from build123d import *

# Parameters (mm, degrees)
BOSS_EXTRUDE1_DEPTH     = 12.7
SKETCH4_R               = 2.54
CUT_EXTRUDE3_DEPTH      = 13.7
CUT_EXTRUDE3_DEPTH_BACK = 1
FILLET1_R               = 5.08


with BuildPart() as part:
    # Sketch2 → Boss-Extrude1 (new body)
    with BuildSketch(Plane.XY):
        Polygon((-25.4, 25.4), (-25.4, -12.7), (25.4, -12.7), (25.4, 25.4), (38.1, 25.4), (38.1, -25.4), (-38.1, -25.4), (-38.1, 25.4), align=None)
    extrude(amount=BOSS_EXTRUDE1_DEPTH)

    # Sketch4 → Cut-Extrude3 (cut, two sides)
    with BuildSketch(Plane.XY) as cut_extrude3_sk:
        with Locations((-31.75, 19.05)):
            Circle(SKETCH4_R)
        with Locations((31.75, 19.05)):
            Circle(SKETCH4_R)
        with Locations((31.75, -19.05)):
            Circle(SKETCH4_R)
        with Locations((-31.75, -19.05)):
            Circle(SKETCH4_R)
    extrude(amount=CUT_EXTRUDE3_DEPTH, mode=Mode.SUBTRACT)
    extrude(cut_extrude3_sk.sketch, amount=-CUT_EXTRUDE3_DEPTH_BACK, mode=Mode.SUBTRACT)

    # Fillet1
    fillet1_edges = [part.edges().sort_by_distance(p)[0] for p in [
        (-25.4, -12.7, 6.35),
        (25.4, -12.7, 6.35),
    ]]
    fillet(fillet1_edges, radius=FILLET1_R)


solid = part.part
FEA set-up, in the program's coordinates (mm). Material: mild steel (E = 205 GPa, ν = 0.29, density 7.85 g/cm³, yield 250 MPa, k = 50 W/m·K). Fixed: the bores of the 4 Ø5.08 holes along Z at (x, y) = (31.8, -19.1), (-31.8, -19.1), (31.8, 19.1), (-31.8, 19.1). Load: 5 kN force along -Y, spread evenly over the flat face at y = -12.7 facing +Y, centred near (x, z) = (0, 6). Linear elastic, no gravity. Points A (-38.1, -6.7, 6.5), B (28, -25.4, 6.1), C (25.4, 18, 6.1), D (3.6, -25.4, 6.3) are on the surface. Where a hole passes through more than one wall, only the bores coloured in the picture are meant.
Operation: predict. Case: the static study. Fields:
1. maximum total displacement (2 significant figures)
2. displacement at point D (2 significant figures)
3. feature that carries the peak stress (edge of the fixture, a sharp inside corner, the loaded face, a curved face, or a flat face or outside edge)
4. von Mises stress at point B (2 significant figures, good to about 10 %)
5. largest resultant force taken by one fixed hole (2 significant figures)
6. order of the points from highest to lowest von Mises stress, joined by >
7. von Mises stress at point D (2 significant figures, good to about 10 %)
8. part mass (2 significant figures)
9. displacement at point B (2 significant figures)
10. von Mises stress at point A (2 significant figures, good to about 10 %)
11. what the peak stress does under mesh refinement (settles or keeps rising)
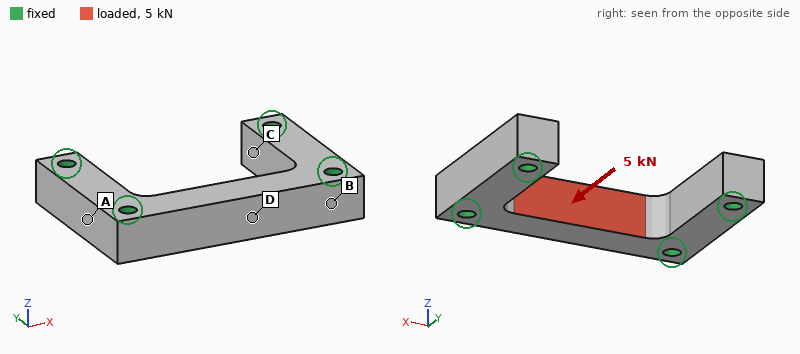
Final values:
14 µm
13 µm
edge of the fixture
44 MPa
2.0 kN
D > B > A > C
56 MPa
190 g
2.3 µm
21 MPa
keeps rising
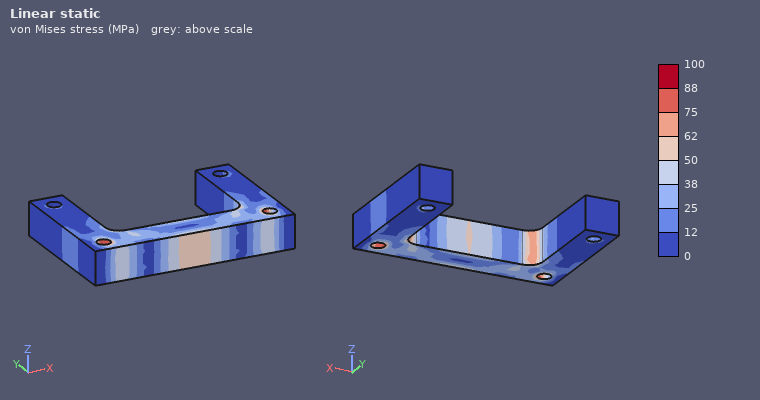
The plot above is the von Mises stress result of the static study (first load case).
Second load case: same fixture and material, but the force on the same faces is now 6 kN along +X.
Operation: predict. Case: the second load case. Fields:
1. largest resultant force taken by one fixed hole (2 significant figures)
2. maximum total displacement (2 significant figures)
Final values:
3.1 kN
2.9 µm
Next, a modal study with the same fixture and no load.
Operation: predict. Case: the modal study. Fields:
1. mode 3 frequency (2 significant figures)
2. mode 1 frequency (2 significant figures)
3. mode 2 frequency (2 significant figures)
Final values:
25 kHz
14 kHz
14 kHz
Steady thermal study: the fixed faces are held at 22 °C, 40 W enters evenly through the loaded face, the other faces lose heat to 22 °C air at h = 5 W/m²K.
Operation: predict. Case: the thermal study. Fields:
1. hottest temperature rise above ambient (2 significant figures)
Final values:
54 K
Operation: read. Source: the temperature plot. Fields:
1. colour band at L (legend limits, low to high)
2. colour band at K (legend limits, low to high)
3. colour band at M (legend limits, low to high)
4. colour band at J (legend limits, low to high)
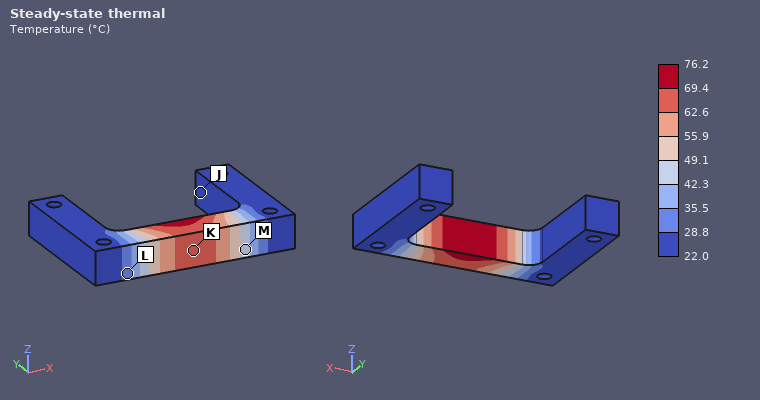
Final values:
28.8 to 35.5 °C
62.6 to 69.4 °C
42.3 to 49.1 °C
22.0 to 28.8 °C
